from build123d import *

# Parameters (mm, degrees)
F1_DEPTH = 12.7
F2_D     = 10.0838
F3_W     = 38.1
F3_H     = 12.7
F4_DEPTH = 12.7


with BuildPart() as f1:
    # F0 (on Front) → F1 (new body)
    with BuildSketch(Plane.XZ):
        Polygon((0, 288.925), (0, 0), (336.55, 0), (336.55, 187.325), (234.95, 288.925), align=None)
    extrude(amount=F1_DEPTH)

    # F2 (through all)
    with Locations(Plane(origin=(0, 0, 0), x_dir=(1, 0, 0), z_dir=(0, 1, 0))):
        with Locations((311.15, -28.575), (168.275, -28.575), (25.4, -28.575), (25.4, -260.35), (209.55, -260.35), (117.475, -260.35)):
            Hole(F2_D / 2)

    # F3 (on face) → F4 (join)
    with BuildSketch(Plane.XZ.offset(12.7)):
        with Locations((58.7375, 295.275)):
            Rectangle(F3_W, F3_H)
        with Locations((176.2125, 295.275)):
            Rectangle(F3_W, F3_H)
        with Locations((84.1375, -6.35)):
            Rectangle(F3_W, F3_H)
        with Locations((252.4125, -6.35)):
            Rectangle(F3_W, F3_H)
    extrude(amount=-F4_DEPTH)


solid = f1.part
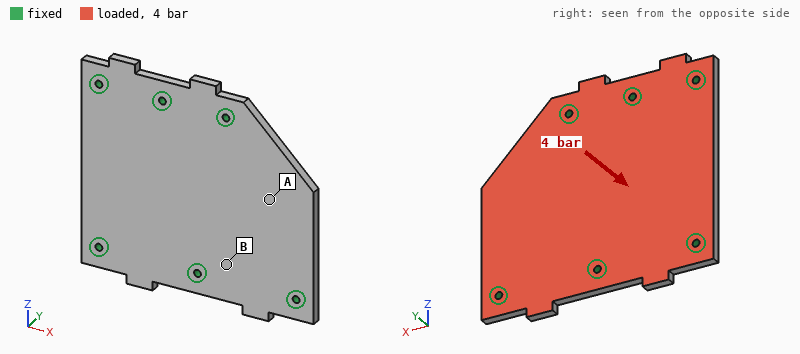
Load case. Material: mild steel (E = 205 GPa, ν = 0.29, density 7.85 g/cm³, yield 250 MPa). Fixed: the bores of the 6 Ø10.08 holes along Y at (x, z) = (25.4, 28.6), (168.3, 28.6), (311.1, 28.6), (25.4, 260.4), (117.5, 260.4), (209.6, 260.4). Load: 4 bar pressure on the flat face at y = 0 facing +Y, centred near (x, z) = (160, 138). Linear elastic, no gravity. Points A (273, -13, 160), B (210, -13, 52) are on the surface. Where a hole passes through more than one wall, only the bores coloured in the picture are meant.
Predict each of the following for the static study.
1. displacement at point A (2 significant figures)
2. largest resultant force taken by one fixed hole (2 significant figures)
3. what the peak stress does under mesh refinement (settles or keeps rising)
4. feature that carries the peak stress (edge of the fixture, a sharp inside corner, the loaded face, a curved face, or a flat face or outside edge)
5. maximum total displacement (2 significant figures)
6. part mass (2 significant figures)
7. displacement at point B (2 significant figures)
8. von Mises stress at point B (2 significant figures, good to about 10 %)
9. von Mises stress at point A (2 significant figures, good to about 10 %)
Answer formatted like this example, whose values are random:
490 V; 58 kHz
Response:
0.18 mm; 8.3 kN; keeps rising; edge of the fixture; 0.26 mm; 9.3 kg; 0.042 mm; 18 MPa; 44 MPa
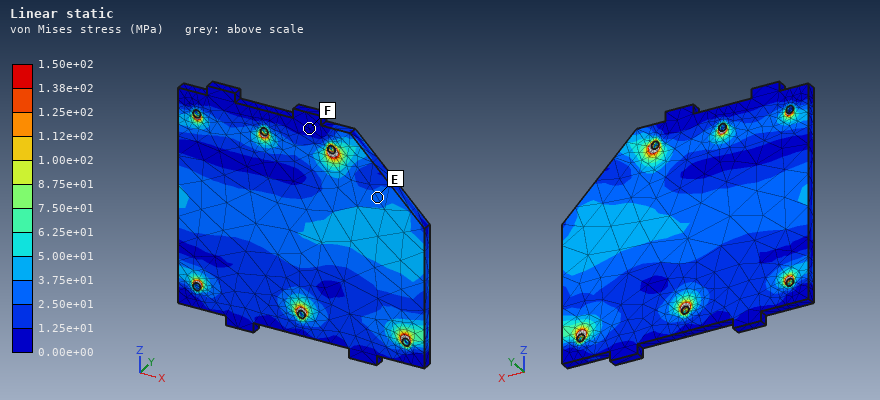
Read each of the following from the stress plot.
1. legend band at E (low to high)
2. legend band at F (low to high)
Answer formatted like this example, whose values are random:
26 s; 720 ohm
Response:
2.50e+01 to 3.75e+01 MPa; 0.00e+00 to 1.25e+01 MPa
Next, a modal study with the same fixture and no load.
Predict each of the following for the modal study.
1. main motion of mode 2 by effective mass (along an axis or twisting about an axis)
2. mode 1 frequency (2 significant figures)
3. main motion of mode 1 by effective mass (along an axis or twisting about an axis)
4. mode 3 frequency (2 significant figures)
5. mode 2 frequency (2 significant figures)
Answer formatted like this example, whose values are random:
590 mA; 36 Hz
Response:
along Y; 830 Hz; along Y; 1500 Hz; 1100 Hz
